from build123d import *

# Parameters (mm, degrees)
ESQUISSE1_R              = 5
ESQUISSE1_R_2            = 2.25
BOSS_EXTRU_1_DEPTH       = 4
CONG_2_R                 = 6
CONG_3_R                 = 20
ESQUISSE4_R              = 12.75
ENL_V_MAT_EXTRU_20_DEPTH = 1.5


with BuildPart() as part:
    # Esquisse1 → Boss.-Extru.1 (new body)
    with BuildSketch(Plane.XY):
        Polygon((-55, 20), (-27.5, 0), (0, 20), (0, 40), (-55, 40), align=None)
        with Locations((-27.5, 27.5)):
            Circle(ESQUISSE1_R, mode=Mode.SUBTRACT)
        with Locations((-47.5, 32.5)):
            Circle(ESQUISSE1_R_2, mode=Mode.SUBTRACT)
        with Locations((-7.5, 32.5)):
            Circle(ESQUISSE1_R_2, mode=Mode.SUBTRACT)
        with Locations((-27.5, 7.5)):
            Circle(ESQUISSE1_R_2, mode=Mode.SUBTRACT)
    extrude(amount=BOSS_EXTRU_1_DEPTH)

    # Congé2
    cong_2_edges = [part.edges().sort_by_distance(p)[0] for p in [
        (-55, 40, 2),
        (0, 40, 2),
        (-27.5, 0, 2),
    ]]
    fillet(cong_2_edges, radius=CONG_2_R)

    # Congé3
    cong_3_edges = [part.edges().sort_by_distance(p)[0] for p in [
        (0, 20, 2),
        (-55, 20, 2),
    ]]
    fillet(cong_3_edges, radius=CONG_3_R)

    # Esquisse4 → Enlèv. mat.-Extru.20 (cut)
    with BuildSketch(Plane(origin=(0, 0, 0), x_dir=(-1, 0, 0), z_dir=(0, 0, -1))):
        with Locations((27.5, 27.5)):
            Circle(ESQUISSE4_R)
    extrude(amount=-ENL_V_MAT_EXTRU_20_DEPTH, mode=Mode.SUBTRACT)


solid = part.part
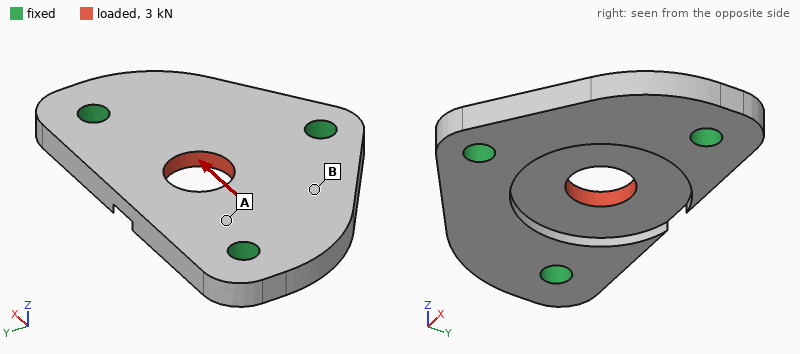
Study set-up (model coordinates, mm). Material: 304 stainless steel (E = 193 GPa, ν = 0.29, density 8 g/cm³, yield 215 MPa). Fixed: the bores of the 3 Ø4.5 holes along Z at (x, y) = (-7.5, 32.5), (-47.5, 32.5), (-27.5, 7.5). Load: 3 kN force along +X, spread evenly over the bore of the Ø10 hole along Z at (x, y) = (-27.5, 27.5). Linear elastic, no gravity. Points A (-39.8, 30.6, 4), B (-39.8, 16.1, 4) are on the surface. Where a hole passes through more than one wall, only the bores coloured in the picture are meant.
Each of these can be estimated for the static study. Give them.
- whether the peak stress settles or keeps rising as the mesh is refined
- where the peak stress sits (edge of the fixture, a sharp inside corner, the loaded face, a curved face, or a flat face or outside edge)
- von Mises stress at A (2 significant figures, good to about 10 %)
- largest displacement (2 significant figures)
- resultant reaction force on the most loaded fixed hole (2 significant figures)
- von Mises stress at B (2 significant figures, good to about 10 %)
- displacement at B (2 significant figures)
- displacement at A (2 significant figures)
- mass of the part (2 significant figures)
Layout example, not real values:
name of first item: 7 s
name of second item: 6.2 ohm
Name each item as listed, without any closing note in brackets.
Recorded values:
whether the peak stress settles or keeps rising as the mesh is refined: keeps rising
where the peak stress sits: edge of the fixture
von Mises stress at A: 35 MPa
largest displacement: 3.4 µm
resultant reaction force on the most loaded fixed hole: 1.1 kN
von Mises stress at B: 9.7 MPa
displacement at B: 1.7 µm
displacement at A: 1.4 µm
mass of the part: 42 g
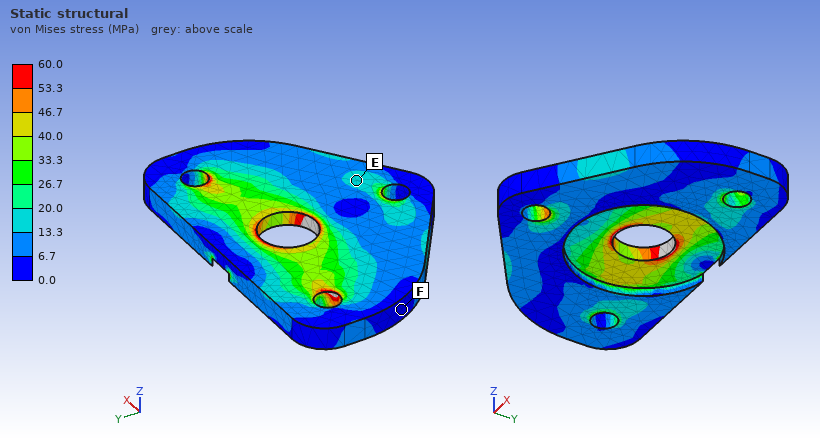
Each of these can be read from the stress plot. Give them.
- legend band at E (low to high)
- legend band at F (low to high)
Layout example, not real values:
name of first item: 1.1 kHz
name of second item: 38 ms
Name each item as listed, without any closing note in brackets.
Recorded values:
legend band at E: 13.3 to 20.0 MPa
legend band at F: 0.0 to 6.7 MPa
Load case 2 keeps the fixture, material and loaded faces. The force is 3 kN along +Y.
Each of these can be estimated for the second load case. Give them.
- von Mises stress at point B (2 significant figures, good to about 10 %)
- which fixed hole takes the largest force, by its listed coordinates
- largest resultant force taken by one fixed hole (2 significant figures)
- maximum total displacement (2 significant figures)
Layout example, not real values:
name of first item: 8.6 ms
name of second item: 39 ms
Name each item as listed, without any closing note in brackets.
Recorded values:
von Mises stress at point B: 12 MPa
which fixed hole takes the largest force, by its listed coordinates: (-27.5, 7.5)
largest resultant force taken by one fixed hole: 1.3 kN
maximum total displacement: 6.8 µm
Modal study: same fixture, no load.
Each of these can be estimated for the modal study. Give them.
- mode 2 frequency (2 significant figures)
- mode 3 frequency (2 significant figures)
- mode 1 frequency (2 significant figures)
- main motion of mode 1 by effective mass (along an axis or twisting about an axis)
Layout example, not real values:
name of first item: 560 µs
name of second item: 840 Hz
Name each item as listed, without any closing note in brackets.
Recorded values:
mode 2 frequency: 16 kHz
mode 3 frequency: 17 kHz
mode 1 frequency: 14 kHz
main motion of mode 1 by effective mass: along Z
